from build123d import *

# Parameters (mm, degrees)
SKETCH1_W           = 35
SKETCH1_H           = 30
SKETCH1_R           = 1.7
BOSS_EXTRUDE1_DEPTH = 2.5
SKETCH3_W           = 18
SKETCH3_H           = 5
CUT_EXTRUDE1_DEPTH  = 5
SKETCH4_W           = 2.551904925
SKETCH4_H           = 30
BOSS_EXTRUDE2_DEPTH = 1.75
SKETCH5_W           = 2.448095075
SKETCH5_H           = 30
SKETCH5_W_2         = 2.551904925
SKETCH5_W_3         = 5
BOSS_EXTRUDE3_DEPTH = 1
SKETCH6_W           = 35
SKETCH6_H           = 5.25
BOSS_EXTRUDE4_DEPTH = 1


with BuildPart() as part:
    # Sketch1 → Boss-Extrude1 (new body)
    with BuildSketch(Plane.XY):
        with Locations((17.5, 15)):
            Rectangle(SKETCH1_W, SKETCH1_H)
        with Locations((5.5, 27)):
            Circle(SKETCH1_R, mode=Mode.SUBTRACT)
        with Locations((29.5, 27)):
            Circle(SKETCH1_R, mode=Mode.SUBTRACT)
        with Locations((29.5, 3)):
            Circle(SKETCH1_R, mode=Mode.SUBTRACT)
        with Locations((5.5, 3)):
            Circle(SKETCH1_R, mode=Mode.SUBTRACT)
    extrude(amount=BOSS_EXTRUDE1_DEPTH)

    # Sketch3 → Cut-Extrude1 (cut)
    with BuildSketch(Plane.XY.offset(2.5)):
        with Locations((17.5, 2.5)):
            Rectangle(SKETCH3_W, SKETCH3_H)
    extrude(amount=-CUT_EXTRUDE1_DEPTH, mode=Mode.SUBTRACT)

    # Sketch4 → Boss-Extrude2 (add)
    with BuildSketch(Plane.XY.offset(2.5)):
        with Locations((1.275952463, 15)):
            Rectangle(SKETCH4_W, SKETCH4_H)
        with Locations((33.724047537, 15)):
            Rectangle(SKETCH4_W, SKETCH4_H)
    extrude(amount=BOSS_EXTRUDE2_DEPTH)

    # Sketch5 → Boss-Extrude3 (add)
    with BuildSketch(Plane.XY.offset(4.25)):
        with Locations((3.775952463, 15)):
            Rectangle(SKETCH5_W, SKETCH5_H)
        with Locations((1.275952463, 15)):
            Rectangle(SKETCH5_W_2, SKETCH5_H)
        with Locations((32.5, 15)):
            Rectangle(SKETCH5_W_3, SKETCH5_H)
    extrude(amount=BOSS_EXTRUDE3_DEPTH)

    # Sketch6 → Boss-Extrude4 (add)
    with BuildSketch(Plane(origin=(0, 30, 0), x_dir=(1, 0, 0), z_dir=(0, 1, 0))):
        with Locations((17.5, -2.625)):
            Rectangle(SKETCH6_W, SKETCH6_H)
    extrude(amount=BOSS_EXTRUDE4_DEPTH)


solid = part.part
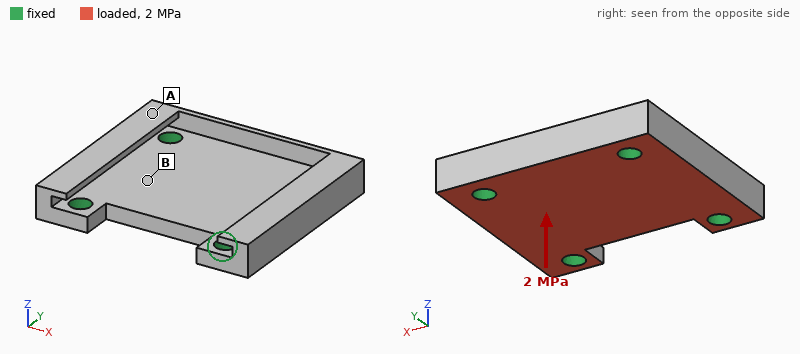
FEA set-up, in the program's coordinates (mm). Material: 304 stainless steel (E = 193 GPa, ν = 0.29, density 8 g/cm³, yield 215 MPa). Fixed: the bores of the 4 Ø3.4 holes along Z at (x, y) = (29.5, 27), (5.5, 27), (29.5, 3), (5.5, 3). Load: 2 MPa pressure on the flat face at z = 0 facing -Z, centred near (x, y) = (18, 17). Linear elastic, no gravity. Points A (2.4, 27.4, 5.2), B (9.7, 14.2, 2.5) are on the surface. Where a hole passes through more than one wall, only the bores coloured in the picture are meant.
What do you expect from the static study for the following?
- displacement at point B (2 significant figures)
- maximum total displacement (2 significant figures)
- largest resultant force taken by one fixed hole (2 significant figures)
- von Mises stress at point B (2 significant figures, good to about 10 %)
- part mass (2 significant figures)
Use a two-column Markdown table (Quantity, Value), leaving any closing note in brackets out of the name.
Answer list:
| Quantity | Value |
|---|---|
| displacement at point B | 9.7 µm |
| maximum total displacement | 14 µm |
| largest resultant force taken by one fixed hole | 550 N |
| von Mises stress at point B | 36 MPa |
| part mass | 24 g |
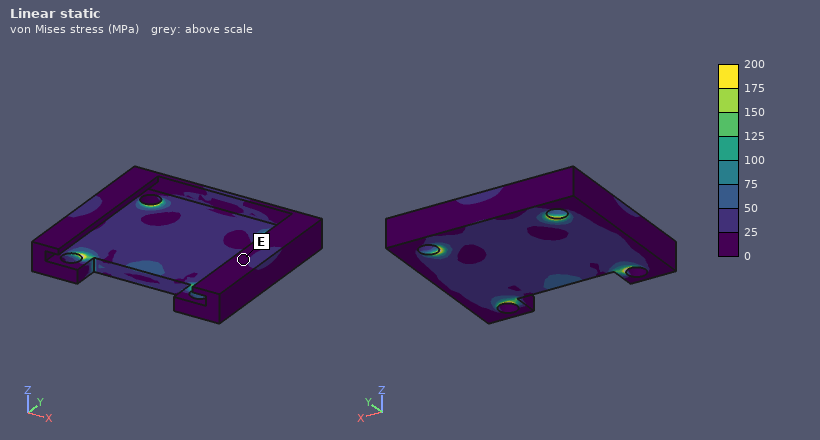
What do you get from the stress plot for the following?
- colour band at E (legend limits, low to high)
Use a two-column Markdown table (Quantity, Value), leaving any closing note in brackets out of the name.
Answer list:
| Quantity | Value |
|---|---|
| colour band at E | 0 to 25 MPa |
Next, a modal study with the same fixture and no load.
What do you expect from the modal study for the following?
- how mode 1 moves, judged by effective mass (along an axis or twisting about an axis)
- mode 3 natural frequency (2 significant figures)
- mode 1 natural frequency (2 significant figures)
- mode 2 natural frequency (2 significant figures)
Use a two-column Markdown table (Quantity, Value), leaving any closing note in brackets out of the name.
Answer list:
| Quantity | Value |
|---|---|
| how mode 1 moves, judged by effective mass | along Z |
| mode 3 natural frequency | 26 kHz |
| mode 1 natural frequency | 16 kHz |
| mode 2 natural frequency | 26 kHz |
